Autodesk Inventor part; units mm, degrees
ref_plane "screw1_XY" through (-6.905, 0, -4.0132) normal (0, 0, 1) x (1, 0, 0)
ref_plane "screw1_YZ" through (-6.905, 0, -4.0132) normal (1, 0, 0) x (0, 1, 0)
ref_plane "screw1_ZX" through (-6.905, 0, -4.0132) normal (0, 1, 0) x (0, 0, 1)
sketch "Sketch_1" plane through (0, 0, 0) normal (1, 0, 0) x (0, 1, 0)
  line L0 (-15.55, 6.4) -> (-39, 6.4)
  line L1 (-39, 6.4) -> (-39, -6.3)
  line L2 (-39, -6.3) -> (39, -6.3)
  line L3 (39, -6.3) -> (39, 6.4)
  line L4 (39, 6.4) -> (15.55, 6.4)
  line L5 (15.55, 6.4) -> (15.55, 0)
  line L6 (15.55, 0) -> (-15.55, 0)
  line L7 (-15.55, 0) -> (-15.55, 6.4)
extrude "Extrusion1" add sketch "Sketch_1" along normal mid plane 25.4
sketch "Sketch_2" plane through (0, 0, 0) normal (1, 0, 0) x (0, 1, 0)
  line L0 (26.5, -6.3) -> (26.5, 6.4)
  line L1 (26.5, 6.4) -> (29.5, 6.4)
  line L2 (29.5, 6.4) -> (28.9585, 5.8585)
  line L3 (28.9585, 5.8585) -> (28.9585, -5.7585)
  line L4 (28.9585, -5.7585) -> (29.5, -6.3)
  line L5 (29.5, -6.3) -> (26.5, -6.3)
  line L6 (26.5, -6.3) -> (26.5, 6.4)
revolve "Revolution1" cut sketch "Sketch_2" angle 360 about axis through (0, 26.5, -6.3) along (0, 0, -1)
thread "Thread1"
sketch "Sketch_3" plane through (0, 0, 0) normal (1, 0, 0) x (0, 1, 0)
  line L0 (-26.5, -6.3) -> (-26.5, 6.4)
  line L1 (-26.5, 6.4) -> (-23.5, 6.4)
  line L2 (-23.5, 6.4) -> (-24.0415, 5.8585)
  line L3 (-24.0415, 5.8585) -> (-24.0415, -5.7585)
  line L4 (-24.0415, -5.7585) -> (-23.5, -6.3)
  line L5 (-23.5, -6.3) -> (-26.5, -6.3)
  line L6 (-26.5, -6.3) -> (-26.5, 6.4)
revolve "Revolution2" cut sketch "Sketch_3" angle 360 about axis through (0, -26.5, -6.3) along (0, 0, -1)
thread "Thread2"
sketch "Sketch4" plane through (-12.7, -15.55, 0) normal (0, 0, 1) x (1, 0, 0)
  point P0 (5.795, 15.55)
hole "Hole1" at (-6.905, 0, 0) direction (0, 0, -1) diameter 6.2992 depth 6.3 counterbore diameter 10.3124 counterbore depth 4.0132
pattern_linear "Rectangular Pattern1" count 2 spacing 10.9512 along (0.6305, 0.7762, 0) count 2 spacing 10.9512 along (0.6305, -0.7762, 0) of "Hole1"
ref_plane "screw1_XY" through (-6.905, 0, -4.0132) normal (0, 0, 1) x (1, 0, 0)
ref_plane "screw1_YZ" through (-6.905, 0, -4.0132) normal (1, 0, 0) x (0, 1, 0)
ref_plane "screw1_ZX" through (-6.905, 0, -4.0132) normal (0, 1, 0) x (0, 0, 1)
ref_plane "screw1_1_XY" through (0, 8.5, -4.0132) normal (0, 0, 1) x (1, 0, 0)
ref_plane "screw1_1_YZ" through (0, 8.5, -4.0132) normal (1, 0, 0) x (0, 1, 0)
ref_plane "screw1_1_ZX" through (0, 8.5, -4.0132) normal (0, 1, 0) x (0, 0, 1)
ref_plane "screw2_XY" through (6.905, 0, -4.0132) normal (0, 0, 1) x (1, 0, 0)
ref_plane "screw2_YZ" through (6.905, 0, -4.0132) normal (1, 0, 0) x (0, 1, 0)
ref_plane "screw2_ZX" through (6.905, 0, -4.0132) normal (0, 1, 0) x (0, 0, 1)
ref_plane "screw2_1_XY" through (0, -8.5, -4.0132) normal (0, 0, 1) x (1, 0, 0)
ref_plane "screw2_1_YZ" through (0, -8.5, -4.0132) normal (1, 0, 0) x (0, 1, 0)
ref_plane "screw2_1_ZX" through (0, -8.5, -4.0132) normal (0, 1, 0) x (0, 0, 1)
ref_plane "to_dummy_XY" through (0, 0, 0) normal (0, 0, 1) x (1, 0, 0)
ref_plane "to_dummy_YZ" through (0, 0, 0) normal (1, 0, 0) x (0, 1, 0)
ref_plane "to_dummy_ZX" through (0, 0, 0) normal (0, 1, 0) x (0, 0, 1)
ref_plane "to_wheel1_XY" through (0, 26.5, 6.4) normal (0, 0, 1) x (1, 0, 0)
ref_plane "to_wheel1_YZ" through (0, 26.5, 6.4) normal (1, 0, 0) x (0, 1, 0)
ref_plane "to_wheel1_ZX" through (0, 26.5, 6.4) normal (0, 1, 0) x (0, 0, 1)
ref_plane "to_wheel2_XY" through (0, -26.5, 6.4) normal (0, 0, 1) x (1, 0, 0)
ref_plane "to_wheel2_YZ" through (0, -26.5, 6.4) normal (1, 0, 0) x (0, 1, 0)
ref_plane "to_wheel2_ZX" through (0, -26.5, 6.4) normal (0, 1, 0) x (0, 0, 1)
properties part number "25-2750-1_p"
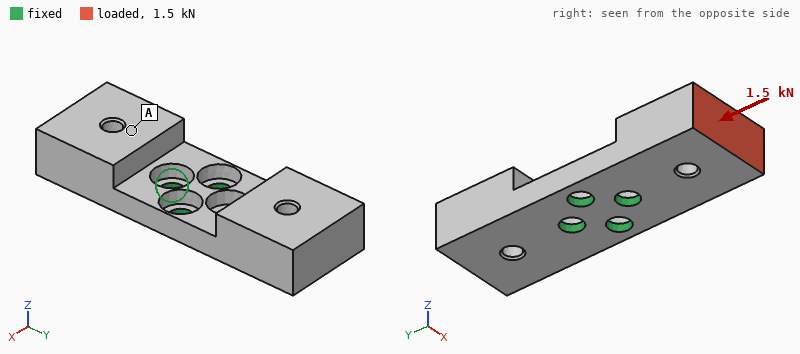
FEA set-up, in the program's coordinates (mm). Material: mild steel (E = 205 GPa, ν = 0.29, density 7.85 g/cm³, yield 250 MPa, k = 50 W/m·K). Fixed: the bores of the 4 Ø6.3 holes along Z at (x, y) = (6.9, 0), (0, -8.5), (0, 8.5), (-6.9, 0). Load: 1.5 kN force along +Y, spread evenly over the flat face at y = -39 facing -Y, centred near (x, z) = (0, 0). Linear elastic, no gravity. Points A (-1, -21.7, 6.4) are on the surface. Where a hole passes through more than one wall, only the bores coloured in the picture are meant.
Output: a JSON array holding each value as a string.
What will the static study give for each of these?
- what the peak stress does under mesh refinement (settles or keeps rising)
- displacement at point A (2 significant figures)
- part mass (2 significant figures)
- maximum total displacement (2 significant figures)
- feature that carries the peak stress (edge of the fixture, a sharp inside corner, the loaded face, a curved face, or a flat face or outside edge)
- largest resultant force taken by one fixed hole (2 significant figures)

["keeps rising", "15 µm", "140 g", "28 µm", "edge of the fixture", "700 N"]
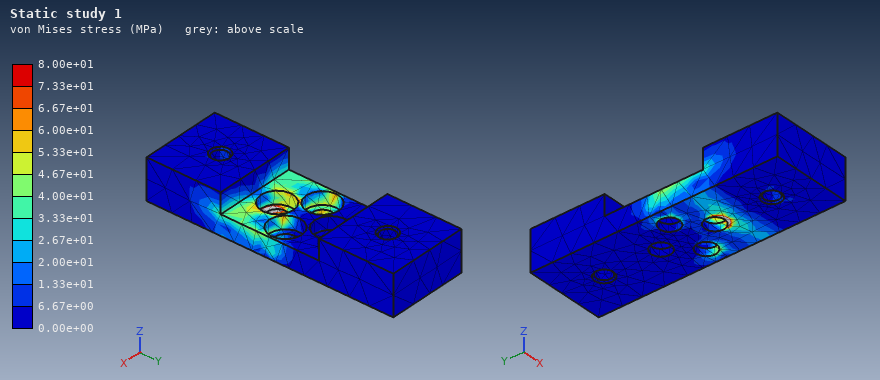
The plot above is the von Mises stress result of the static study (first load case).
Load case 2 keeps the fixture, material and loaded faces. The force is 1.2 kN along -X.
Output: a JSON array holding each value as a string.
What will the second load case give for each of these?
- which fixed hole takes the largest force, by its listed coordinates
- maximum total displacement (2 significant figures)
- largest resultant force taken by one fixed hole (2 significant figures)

["(0, -8.5)", "18 µm", "1.7 kN"]
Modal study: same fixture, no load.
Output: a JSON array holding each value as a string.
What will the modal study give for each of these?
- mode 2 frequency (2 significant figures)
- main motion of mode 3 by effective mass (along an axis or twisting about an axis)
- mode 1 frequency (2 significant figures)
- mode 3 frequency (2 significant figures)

["3000 Hz", "twisting about Z", "2900 Hz", "7000 Hz"]
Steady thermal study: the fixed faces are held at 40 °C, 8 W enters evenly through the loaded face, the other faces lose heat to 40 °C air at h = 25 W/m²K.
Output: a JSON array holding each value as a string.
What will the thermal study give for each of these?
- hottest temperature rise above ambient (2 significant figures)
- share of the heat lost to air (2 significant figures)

["24 K", "13 %"]
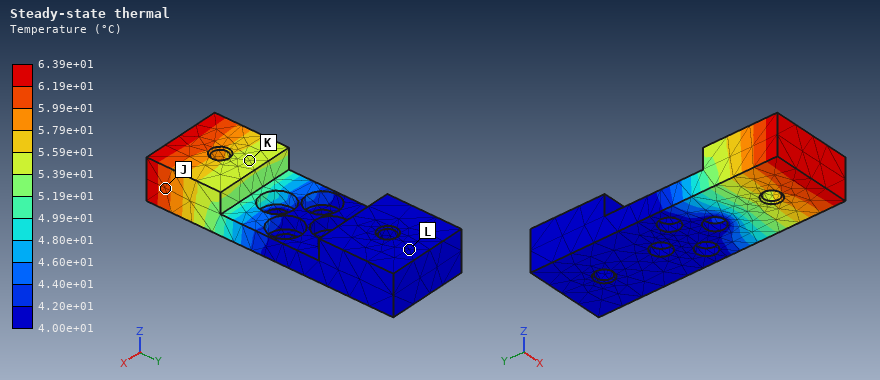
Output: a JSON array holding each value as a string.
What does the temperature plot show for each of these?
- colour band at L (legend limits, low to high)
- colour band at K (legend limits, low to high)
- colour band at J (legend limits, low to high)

["4.00e+01 to 4.20e+01 °C", "5.39e+01 to 5.59e+01 °C", "5.99e+01 to 6.19e+01 °C"]
